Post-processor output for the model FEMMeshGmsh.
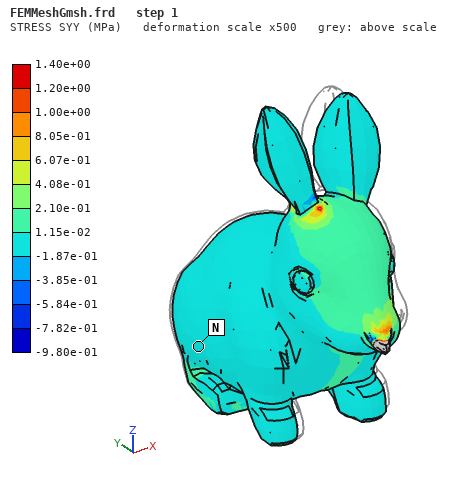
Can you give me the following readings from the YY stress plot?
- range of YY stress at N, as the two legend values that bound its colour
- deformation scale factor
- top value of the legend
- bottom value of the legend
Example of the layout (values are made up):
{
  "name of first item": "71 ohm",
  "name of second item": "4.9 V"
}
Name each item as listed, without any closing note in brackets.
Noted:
{
  "range of YY stress at N, as the two legend values that bound its colour": "-1.87e-01 to 1.15e-02 MPa",
  "deformation scale factor": "500",
  "top value of the legend": "1.40e+00 MPa",
  "bottom value of the legend": "-9.80e-01 MPa"
}
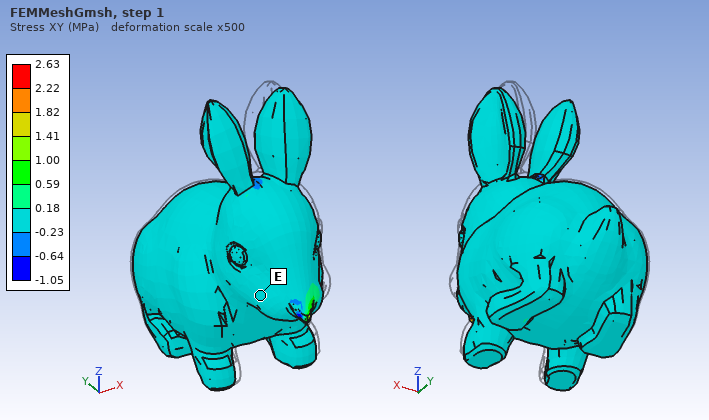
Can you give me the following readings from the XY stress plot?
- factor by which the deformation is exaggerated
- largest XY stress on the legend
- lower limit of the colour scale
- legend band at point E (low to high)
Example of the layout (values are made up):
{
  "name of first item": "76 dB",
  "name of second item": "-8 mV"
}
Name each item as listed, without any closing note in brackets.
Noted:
{
  "factor by which the deformation is exaggerated": "500",
  "largest XY stress on the legend": "2.63 MPa",
  "lower limit of the colour scale": "-1.05 MPa",
  "legend band at point E": "-0.23 to 0.18 MPa"
}
